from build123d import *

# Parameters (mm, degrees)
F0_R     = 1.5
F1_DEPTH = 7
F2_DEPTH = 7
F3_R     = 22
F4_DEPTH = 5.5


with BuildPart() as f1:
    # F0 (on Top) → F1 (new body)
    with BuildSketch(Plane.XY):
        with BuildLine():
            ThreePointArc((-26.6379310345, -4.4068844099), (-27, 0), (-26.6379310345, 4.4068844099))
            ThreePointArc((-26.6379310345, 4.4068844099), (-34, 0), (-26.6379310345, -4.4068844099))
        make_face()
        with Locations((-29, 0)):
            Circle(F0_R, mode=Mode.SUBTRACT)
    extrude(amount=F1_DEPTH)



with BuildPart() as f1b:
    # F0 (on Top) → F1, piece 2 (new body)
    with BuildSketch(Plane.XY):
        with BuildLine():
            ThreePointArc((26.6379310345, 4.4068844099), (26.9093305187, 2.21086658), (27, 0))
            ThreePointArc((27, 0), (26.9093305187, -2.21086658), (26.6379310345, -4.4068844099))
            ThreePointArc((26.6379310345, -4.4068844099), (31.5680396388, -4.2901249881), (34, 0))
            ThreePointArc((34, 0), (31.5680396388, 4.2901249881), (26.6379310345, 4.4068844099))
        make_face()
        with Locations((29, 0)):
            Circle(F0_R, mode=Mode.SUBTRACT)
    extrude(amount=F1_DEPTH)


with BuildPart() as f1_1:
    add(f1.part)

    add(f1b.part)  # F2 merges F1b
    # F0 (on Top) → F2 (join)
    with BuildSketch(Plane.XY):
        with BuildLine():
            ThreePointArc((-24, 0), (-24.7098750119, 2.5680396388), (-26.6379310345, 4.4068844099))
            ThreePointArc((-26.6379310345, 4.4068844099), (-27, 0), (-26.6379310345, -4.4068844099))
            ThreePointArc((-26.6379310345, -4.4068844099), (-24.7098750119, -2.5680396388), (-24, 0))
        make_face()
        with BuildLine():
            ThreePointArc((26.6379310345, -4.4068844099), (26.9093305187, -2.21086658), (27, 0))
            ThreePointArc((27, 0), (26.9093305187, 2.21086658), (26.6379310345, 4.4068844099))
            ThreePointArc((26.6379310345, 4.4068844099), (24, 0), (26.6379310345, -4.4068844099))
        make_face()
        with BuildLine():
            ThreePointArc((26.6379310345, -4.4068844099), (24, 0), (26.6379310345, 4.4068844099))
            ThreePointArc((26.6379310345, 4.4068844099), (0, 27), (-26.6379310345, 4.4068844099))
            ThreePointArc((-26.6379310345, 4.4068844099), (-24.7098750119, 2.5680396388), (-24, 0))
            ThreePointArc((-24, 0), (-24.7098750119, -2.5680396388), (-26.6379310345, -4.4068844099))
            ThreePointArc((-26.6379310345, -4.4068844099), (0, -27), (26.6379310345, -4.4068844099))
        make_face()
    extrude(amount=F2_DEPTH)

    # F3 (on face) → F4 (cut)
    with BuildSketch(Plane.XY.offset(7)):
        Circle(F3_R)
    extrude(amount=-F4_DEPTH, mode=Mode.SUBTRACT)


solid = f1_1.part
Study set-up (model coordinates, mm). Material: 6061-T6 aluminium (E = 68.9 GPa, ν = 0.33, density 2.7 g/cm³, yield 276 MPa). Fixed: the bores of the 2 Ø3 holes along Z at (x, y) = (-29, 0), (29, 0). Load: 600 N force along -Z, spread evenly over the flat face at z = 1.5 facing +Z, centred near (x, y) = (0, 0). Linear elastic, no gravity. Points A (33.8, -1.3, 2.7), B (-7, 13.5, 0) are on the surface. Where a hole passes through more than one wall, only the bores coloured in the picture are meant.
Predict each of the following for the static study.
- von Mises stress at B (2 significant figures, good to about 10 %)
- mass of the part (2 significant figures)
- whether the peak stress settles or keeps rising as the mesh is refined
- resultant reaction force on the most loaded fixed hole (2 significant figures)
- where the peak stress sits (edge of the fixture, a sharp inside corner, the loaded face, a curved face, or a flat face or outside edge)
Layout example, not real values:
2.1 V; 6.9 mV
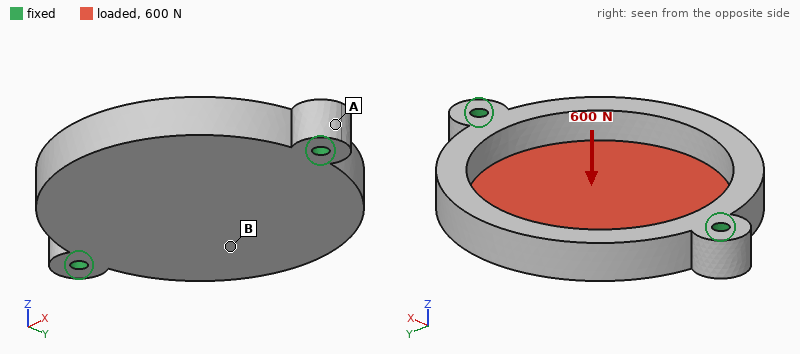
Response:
26 MPa; 23 g; keeps rising; 370 N; edge of the fixture
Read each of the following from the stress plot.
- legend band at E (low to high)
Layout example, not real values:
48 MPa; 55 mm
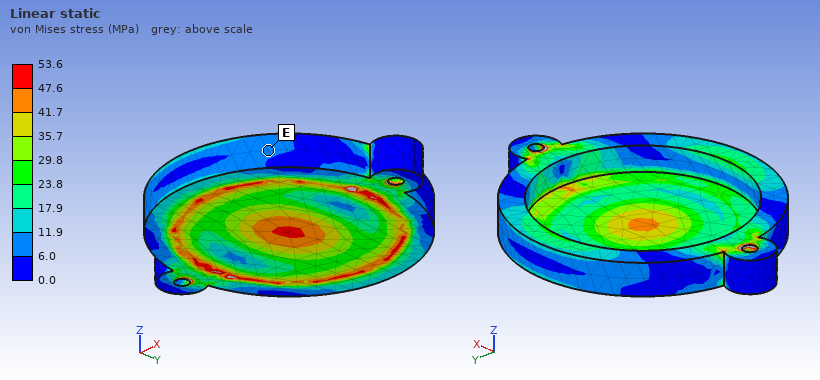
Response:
6.0 to 11.9 MPa
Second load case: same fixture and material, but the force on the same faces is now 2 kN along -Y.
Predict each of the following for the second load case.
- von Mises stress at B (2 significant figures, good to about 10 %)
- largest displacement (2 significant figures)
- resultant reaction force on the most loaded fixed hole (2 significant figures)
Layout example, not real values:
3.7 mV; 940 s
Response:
13 MPa; 37 µm; 1.0 kN
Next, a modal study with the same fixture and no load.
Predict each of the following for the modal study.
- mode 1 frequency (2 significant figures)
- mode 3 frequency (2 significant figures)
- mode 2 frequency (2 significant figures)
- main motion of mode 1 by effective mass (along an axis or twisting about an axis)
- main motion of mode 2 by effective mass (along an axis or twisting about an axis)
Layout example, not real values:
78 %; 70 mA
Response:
4100 Hz; 7400 Hz; 5000 Hz; twisting about X; along Z
